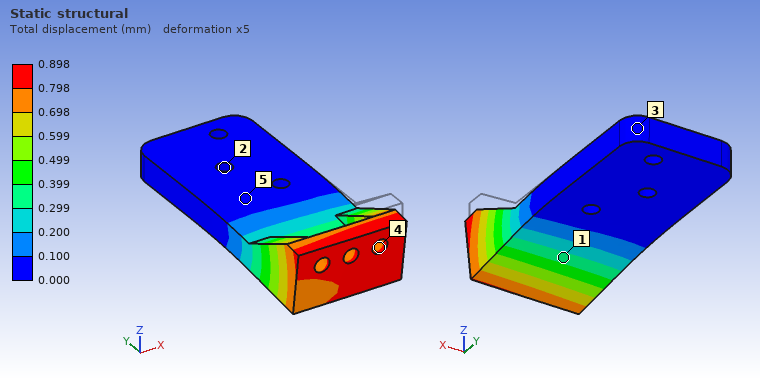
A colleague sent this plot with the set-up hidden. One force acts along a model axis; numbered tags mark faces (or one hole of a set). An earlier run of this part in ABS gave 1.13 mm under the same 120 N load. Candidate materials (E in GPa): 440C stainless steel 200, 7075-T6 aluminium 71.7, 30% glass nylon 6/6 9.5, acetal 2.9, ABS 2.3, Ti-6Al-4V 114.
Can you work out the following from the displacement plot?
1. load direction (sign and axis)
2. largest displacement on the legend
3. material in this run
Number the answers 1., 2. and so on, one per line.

1. -Z
2. 0.898 mm
3. acetal
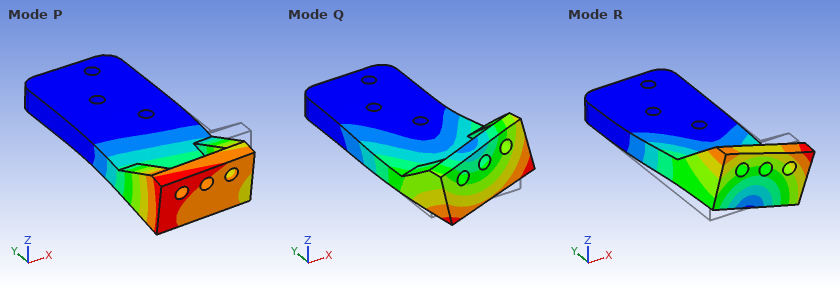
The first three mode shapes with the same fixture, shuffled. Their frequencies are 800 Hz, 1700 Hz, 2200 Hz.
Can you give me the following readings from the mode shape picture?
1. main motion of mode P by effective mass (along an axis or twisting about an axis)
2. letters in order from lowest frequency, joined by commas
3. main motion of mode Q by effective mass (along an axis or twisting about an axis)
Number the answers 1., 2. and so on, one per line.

1. along Z
2. P, R, Q
3. along X
